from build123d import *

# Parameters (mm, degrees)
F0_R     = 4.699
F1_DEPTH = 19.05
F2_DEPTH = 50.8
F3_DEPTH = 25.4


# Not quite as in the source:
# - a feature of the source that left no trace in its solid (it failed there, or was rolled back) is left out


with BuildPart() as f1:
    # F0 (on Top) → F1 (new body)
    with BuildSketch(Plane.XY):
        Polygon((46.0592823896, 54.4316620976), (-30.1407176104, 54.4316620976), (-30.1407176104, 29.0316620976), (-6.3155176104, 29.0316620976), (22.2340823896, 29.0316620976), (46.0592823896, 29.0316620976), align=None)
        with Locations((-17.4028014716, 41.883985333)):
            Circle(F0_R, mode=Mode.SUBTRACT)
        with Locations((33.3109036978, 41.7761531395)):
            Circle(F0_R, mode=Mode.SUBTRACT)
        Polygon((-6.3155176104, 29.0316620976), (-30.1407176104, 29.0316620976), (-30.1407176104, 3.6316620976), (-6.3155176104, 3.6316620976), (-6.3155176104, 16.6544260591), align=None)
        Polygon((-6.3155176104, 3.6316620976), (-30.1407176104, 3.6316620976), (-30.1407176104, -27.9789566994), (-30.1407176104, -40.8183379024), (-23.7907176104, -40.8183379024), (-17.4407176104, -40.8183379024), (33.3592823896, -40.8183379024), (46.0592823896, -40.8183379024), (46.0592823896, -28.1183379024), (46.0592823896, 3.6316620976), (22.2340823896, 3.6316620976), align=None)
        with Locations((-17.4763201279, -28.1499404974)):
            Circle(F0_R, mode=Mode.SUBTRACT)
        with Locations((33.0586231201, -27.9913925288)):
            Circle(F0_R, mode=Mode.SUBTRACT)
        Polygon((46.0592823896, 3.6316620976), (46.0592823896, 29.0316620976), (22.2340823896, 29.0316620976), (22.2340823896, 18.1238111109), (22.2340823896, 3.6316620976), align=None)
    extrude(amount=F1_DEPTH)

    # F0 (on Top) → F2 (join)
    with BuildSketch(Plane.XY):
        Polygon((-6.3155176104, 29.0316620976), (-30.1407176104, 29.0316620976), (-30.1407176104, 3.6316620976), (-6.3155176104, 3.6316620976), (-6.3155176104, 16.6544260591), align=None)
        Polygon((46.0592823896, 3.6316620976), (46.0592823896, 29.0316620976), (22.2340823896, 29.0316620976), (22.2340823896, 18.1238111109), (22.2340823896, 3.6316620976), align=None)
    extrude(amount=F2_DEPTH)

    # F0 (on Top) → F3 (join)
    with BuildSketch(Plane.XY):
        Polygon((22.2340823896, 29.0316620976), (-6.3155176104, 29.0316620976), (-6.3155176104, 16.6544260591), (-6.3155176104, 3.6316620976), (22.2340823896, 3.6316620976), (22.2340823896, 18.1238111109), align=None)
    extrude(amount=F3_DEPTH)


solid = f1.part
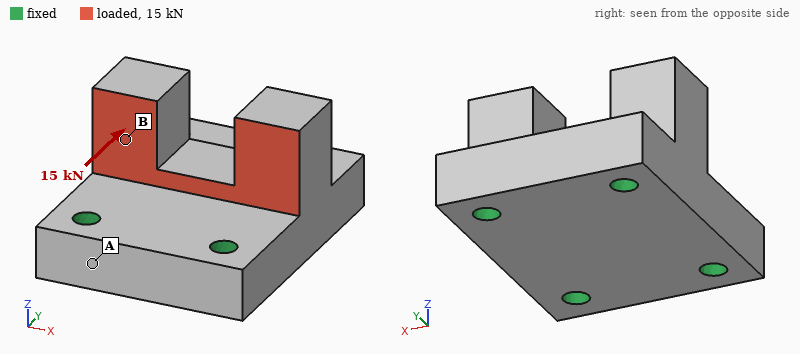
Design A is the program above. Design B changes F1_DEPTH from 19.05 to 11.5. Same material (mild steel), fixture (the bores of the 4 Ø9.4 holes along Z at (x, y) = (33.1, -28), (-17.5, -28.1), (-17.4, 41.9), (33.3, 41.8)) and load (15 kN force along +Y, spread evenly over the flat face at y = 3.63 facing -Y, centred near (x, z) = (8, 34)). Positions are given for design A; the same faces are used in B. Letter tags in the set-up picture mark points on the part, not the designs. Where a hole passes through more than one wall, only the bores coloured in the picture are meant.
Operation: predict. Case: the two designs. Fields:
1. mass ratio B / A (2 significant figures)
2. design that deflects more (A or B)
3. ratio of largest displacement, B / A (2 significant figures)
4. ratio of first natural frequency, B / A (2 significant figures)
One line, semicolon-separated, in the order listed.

0.78; B; 2.0; 0.65
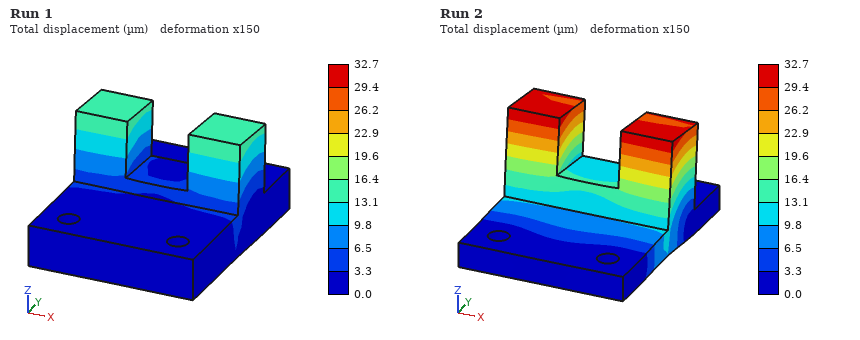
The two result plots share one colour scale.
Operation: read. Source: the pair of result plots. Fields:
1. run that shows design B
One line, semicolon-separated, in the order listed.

Run 2
